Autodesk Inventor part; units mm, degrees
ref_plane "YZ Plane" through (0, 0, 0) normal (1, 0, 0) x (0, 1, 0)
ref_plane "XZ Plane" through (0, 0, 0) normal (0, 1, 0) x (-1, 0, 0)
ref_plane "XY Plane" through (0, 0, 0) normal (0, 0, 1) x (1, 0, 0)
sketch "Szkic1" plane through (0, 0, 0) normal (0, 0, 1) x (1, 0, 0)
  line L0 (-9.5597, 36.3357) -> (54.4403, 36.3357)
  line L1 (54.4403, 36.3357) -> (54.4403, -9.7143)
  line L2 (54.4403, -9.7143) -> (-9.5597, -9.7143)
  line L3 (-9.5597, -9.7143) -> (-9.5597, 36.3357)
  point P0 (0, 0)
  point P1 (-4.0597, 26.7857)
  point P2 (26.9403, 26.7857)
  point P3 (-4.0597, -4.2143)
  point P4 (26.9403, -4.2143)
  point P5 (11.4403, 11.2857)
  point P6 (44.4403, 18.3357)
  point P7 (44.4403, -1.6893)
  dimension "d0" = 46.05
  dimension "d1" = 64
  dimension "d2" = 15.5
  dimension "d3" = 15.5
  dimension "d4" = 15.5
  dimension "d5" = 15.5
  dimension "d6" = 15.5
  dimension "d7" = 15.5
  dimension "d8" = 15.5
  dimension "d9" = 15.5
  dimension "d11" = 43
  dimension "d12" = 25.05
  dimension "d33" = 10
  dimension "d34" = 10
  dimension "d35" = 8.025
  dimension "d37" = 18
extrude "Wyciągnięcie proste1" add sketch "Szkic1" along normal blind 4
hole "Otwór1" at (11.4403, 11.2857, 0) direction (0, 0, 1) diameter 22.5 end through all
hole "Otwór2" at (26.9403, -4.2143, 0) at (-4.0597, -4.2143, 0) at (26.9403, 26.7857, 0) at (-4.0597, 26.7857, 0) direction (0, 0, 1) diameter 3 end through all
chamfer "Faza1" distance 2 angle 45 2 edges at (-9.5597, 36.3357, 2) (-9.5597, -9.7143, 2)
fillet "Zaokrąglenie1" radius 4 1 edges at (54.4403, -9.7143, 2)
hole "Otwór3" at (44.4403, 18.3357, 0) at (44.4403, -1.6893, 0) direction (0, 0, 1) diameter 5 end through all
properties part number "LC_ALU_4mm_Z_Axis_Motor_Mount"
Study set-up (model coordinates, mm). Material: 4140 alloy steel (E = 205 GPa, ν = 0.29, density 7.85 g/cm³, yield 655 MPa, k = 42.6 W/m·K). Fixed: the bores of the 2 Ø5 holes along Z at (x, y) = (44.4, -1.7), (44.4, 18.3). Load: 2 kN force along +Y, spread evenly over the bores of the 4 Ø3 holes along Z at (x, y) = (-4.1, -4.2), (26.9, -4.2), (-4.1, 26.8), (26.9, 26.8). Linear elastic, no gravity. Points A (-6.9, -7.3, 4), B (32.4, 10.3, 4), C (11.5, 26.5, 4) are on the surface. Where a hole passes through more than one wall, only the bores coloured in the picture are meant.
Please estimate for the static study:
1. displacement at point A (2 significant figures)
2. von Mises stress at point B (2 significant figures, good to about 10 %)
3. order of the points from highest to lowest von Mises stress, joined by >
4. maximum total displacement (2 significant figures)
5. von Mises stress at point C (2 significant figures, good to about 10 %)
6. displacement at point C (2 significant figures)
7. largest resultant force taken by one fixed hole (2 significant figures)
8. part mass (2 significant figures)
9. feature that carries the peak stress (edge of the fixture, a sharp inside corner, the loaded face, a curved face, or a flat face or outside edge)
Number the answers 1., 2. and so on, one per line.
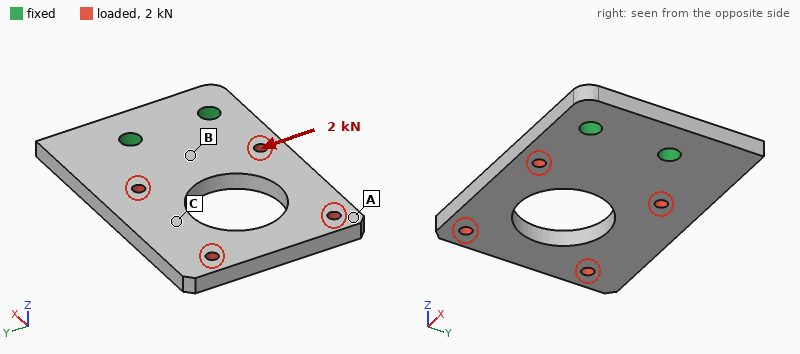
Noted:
1. 32 µm
2. 50 MPa
3. B > C > A
4. 34 µm
5. 25 MPa
6. 19 µm
7. 2.9 kN
8. 78 g
9. edge of the fixture
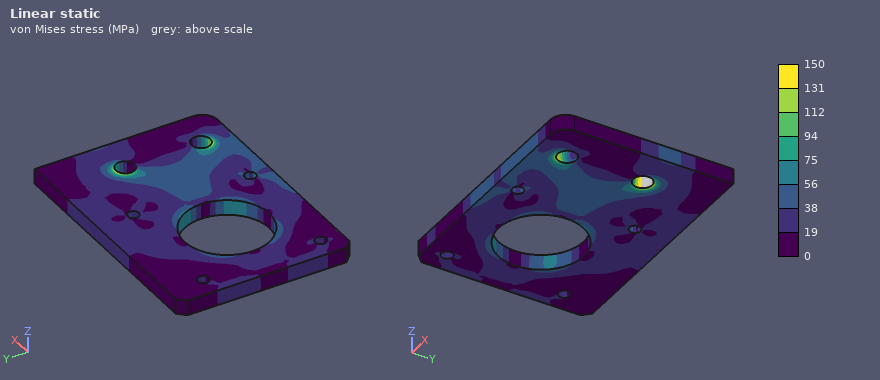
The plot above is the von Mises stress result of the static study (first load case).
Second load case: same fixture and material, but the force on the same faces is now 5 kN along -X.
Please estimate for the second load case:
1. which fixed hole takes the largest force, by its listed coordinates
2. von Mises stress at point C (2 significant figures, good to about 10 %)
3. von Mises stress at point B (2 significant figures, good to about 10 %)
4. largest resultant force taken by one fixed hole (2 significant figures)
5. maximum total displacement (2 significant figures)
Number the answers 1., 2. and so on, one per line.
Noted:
1. (44.4, 18.3)
2. 27 MPa
3. 14 MPa
4. 3.1 kN
5. 10 µm
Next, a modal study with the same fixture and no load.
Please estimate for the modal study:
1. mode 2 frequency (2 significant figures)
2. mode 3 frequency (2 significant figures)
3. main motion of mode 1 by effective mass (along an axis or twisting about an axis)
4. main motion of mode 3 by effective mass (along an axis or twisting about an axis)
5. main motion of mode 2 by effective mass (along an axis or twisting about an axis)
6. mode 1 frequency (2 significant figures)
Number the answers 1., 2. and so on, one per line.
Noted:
1. 2700 Hz
2. 6100 Hz
3. along Z
4. along Z
5. twisting about X
6. 1200 Hz
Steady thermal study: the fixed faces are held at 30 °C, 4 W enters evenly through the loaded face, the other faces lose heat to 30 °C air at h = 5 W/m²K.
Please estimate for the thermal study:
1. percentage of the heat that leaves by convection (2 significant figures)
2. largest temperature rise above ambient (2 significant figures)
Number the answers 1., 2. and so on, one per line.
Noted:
1. 8.1 %
2. 24 K
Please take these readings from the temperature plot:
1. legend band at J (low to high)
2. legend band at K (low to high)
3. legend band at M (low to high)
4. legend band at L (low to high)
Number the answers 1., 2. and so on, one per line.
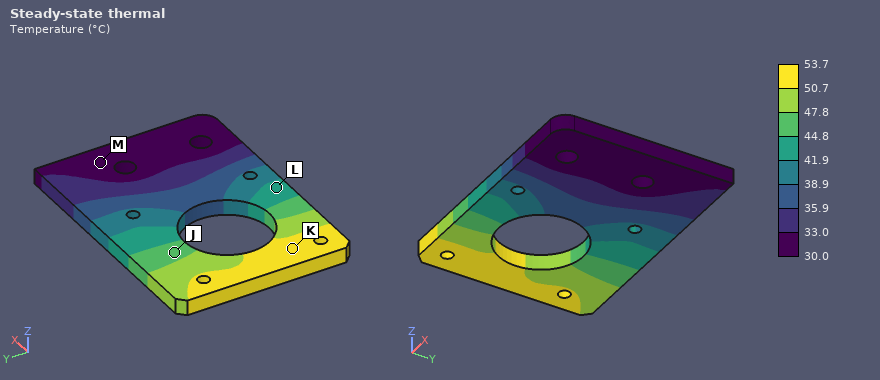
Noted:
1. 44.8 to 47.8 °C
2. 50.7 to 53.7 °C
3. 30.0 to 33.0 °C
4. 41.9 to 44.8 °C
